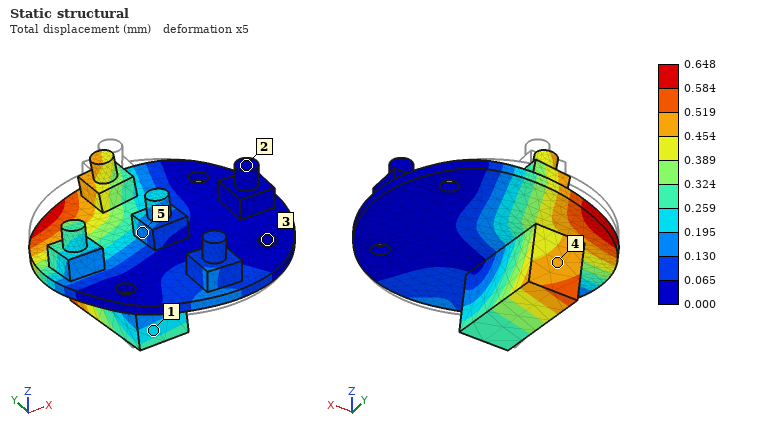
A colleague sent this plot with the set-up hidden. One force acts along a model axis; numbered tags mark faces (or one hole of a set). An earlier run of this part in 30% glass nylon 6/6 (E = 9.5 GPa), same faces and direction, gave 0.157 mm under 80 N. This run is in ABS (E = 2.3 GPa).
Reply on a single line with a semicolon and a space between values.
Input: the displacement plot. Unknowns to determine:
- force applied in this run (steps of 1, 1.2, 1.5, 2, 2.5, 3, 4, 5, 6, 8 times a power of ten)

80 N
